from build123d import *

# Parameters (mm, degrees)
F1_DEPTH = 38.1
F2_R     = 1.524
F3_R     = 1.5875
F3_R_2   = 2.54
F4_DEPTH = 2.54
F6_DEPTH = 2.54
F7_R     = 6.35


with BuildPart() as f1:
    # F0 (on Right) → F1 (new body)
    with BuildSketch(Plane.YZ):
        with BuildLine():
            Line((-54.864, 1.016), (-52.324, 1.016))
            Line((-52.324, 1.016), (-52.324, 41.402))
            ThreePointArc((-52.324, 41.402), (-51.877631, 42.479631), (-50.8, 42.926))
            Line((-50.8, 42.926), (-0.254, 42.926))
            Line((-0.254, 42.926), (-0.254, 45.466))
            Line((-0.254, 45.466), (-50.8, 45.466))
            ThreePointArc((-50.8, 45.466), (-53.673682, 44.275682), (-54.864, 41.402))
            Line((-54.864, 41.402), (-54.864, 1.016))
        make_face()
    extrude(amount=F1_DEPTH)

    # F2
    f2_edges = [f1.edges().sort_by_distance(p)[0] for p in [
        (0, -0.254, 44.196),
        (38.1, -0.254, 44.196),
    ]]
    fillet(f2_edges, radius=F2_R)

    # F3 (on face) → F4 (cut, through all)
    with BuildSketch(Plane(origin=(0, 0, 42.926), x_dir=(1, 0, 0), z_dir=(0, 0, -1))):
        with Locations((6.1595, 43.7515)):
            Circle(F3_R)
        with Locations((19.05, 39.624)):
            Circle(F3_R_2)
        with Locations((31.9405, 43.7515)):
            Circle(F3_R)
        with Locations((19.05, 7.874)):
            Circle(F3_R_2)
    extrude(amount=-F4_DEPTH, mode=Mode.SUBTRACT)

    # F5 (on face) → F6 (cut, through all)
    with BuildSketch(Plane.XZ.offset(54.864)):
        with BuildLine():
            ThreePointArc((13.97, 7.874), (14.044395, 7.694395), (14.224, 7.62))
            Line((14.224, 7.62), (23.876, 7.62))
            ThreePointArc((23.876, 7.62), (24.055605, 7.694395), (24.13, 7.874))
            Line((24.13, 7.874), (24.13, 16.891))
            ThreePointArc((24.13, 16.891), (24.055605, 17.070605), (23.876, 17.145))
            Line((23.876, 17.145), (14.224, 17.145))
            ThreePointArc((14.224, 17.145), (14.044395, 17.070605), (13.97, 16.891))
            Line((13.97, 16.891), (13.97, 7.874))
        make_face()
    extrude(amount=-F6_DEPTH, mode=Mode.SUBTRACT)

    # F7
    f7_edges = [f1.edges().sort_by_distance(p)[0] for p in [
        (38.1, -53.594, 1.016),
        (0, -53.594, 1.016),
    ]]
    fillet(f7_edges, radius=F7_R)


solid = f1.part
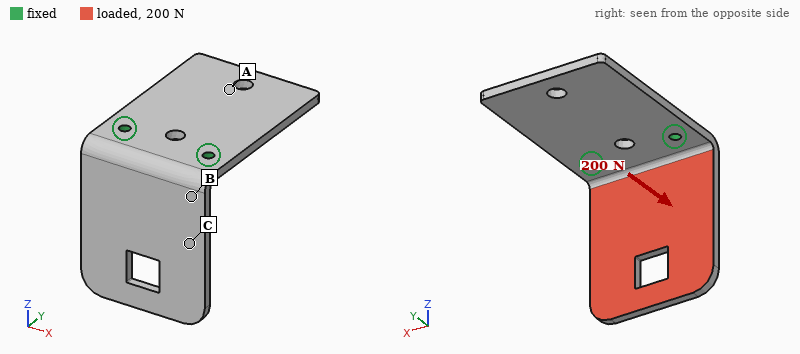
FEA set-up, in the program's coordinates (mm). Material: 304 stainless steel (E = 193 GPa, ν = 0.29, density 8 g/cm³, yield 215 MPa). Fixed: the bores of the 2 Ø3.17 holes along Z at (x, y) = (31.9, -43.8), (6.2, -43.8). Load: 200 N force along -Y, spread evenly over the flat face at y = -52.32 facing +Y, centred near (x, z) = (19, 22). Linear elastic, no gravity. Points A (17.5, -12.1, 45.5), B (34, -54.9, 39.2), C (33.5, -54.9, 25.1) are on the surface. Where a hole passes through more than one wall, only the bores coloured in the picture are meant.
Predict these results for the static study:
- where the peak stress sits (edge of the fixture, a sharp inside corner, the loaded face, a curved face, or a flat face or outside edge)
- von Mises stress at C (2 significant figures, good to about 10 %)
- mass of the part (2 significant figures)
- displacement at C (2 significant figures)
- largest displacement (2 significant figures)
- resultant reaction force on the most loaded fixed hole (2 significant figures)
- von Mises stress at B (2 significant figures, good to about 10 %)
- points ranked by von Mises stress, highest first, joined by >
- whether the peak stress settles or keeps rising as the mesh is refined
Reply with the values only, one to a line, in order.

edge of the fixture
34 MPa
70 g
0.13 mm
0.36 mm
100 N
77 MPa
B > C > A
keeps rising
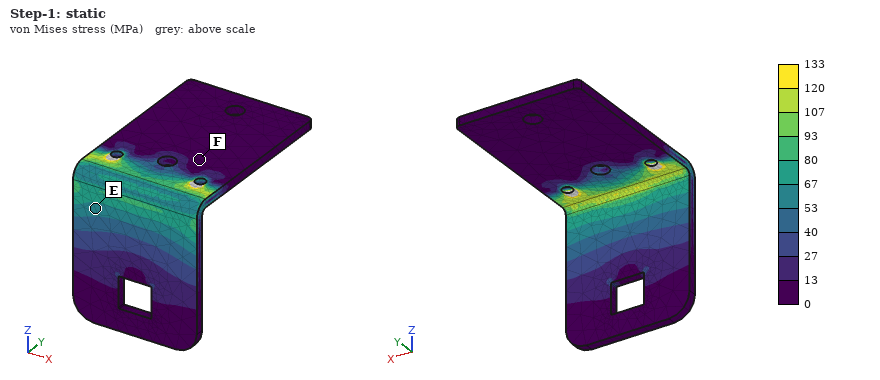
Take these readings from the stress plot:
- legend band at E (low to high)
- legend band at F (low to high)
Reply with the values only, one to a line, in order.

53 to 67 MPa
0 to 13 MPa
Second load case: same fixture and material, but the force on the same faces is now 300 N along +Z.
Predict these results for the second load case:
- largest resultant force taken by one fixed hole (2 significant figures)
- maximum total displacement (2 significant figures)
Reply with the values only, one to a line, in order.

150 N
30 µm
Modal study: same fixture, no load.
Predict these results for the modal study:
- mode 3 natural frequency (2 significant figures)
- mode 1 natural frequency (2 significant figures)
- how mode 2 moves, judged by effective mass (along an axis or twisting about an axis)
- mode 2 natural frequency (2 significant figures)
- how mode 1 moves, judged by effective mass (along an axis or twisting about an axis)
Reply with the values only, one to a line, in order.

2400 Hz
860 Hz
along Z
1100 Hz
along Y
